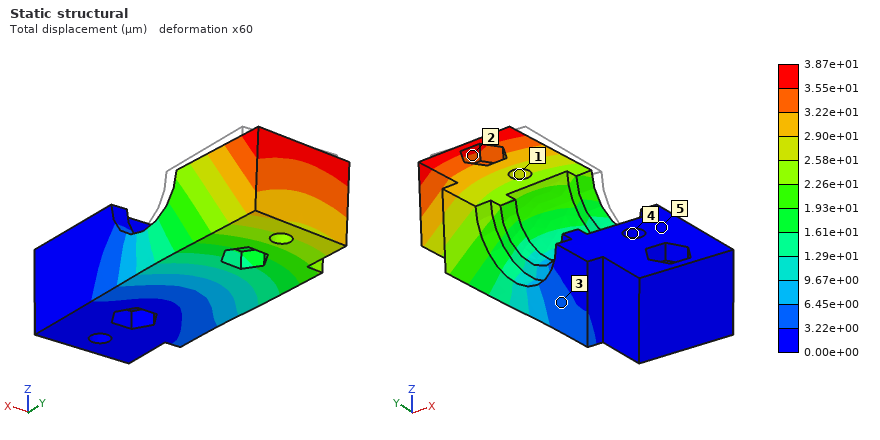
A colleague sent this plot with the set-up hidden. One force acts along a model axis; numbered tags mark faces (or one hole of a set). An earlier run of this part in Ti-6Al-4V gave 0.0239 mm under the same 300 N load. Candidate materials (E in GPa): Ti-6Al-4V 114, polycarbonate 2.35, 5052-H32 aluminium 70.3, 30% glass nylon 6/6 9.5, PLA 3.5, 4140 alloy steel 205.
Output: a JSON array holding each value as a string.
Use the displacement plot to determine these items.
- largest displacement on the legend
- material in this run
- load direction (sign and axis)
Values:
["3.87e+01 µm", "5052-H32 aluminium", "-X"]
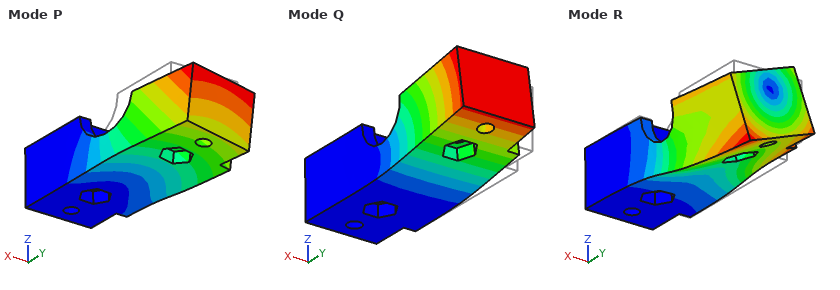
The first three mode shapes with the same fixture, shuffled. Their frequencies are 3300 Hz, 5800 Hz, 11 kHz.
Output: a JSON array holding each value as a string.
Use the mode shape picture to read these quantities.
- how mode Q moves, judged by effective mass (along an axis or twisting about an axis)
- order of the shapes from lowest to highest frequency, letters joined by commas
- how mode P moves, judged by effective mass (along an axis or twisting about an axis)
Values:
["along Z", "Q, P, R", "along X"]
